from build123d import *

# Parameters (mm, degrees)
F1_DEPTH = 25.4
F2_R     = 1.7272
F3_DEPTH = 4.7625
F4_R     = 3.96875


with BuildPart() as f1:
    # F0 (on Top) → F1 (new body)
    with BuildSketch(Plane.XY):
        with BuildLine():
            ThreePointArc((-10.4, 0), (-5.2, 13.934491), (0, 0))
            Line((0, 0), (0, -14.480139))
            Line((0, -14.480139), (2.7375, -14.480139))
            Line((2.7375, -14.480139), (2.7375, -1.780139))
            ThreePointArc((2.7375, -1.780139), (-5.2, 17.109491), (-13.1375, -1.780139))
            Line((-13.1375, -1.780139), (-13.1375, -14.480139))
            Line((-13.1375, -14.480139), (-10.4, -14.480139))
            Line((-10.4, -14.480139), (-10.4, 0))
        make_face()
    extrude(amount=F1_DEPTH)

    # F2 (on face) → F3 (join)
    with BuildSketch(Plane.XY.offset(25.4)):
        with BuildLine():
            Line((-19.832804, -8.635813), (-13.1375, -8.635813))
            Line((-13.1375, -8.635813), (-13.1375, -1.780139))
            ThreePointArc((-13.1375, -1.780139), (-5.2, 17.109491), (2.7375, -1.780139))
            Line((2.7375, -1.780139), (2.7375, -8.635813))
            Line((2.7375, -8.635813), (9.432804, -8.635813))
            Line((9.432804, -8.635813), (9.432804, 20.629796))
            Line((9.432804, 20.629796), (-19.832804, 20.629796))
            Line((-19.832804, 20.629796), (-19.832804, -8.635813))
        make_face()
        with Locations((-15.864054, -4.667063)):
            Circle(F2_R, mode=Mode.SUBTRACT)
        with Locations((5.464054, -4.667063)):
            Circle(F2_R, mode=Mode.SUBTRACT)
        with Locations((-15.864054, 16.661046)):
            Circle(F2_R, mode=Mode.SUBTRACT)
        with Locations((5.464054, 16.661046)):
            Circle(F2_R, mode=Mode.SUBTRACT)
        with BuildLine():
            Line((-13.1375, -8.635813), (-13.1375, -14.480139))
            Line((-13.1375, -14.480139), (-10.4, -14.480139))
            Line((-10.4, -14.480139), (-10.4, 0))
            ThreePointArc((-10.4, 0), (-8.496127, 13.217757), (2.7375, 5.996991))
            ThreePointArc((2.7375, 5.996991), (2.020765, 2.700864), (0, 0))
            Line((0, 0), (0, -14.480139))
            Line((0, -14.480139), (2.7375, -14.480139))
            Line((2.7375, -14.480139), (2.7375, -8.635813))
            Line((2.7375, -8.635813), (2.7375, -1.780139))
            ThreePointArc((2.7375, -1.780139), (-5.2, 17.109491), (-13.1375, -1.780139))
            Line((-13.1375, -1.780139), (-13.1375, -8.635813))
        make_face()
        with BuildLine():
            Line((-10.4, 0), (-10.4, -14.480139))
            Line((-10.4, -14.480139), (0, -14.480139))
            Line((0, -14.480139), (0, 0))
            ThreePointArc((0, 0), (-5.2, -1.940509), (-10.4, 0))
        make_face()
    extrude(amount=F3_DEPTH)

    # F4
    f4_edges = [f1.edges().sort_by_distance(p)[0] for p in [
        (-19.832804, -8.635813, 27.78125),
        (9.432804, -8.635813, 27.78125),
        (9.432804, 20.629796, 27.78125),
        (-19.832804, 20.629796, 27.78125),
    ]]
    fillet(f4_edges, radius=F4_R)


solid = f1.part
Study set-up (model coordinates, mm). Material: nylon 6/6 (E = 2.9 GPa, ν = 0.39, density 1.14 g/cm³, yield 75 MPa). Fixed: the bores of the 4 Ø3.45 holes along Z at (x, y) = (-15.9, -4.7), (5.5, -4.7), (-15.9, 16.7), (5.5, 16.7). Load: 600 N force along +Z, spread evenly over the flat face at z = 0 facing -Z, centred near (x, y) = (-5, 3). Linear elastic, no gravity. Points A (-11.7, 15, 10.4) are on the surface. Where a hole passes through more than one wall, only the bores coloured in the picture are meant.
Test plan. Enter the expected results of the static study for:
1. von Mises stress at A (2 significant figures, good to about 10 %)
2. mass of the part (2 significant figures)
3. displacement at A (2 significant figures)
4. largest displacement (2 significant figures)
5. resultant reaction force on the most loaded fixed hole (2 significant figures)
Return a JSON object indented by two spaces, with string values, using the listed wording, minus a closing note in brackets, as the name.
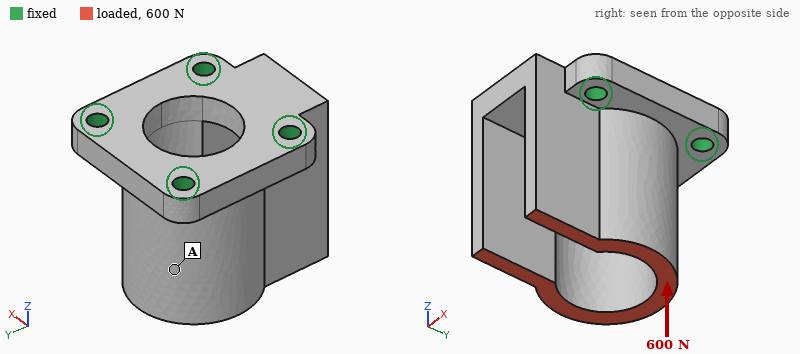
{
  "von Mises stress at A": "2.6 MPa",
  "mass of the part": "10 g",
  "displacement at A": "32 µm",
  "largest displacement": "51 µm",
  "resultant reaction force on the most loaded fixed hole": "190 N"
}
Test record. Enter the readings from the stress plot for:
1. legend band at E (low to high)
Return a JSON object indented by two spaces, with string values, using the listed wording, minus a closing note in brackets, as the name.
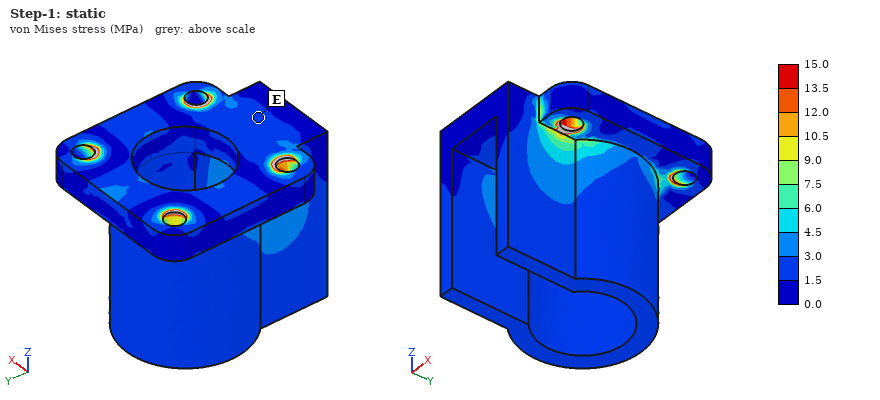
{
  "legend band at E": "1.5 to 3.0 MPa"
}
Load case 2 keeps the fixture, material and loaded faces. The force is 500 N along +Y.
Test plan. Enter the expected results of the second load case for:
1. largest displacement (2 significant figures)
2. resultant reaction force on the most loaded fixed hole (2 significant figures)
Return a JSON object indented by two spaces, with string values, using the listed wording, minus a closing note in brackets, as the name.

{
  "largest displacement": "0.56 mm",
  "resultant reaction force on the most loaded fixed hole": "360 N"
}
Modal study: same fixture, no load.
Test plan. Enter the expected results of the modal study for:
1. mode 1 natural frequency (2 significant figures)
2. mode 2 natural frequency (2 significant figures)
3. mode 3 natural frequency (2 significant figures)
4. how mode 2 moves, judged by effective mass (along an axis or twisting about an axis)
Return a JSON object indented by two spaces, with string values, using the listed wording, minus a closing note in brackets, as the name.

{
  "mode 1 natural frequency": "1800 Hz",
  "mode 2 natural frequency": "1900 Hz",
  "mode 3 natural frequency": "3600 Hz",
  "how mode 2 moves, judged by effective mass": "along X"
}
